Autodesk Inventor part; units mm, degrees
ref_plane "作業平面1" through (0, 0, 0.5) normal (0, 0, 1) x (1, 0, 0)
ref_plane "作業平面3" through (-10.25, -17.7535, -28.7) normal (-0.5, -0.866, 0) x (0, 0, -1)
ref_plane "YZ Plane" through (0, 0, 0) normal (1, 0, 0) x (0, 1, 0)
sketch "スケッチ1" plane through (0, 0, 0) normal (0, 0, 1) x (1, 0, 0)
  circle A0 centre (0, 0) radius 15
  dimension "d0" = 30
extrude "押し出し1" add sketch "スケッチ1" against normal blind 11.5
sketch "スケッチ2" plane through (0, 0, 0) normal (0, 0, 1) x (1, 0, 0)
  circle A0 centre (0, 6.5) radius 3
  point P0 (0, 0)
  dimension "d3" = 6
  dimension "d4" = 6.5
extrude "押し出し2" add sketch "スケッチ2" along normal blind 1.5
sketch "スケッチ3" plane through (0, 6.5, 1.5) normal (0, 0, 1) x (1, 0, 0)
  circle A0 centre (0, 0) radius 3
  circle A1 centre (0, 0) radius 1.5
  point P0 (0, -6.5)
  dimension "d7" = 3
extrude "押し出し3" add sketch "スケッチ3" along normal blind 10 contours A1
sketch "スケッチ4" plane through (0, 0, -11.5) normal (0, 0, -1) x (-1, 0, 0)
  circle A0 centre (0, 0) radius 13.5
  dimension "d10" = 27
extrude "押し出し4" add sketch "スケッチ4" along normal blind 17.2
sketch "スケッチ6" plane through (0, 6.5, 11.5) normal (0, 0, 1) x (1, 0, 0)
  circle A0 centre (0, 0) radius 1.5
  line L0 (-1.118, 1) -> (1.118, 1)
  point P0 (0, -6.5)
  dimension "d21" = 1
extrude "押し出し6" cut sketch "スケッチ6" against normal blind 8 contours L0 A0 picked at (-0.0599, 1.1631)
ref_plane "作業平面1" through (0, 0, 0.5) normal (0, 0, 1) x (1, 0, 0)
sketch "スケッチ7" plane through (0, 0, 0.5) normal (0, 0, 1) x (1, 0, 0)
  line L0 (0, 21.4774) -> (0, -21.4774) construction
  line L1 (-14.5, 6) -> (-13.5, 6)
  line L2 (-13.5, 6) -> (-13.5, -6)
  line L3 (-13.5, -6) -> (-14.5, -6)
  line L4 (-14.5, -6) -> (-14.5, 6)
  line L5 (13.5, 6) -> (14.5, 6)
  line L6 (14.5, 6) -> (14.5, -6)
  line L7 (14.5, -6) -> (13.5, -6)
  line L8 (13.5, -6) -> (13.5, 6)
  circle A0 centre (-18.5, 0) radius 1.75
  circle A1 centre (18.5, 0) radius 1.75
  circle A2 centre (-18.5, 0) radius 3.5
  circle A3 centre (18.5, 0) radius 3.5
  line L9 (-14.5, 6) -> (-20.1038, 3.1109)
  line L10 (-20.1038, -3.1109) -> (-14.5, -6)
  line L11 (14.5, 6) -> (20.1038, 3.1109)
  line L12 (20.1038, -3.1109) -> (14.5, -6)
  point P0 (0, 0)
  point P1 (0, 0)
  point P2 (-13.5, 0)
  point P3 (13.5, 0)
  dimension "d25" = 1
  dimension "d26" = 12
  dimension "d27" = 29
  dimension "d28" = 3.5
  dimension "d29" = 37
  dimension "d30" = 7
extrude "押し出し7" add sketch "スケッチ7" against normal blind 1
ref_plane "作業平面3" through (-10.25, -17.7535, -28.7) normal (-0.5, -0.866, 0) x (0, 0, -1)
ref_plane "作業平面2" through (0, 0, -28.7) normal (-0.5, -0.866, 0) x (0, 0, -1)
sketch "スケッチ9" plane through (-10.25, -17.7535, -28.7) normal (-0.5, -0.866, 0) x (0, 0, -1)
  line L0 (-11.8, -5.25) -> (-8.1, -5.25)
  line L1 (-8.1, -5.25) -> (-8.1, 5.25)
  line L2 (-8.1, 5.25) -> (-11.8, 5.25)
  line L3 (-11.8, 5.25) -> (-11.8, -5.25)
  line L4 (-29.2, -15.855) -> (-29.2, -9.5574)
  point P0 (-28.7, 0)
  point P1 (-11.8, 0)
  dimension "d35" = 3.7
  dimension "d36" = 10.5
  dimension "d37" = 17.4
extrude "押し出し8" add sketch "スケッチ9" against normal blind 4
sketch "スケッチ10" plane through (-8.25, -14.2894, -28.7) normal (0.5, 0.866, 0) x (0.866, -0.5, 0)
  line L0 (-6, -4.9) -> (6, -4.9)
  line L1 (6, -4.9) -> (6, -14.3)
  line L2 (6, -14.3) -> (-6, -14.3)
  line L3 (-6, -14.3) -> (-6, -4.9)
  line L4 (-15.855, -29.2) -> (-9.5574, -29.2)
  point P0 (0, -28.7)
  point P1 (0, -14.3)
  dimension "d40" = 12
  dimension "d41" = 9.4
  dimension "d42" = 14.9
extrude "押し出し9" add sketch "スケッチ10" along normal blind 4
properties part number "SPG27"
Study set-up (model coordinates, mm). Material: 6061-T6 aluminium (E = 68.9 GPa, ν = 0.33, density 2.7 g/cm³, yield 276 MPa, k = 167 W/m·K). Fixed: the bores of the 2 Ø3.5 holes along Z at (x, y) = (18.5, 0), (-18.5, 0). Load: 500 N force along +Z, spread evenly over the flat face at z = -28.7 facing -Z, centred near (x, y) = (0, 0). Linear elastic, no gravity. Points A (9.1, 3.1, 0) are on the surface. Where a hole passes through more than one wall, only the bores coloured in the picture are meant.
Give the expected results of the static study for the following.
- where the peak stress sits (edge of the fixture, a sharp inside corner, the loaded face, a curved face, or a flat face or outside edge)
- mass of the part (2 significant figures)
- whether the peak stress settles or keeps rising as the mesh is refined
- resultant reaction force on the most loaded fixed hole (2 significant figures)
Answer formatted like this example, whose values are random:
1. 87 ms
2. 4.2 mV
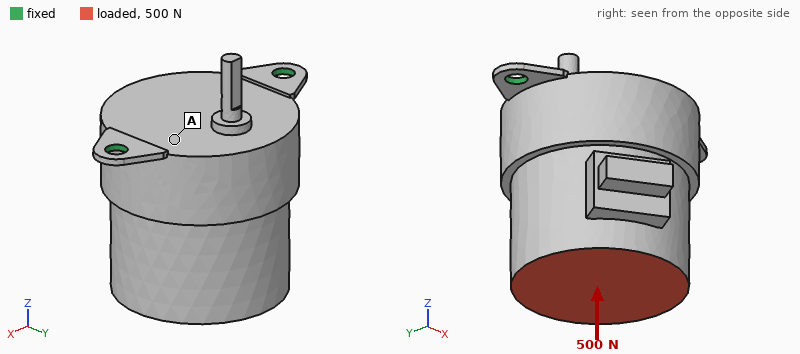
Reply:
1. edge of the fixture
2. 51 g
3. keeps rising
4. 310 N
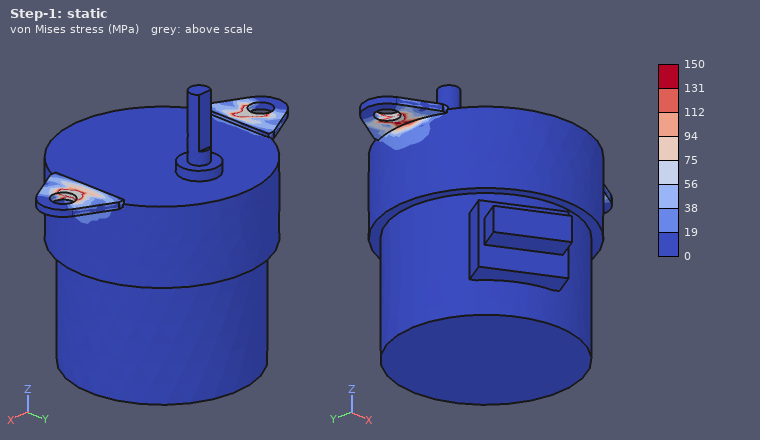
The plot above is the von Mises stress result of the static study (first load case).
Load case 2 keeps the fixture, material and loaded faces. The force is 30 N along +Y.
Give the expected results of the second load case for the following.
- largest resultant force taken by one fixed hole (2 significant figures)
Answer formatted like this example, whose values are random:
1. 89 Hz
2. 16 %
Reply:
1. 15 N
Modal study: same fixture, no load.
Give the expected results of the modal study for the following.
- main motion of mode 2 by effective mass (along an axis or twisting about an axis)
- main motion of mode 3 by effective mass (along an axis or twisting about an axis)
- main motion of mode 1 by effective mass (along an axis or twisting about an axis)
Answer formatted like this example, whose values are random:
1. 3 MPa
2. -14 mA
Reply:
1. along X
2. along Z
3. along Y
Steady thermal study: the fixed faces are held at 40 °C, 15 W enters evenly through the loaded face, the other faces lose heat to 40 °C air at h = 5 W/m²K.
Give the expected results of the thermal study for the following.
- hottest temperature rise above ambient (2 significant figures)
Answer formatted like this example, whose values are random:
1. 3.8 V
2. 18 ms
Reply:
1. 25 K
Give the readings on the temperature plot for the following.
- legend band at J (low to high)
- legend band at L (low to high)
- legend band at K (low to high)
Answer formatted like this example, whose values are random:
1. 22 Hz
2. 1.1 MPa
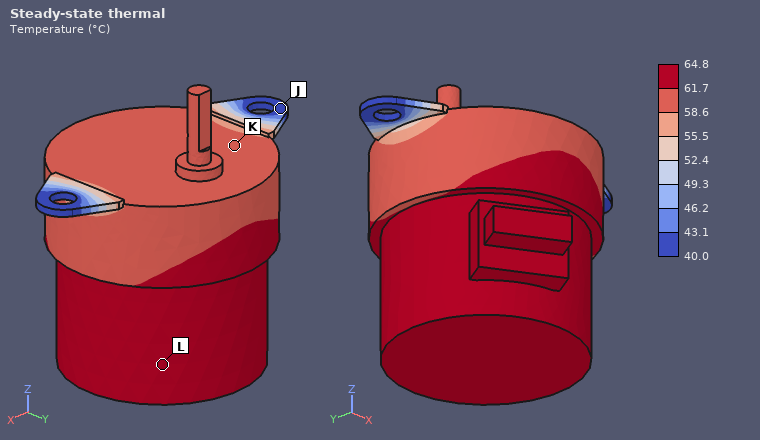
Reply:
1. 40.0 to 43.1 °C
2. 61.7 to 64.8 °C
3. 58.6 to 61.7 °C
